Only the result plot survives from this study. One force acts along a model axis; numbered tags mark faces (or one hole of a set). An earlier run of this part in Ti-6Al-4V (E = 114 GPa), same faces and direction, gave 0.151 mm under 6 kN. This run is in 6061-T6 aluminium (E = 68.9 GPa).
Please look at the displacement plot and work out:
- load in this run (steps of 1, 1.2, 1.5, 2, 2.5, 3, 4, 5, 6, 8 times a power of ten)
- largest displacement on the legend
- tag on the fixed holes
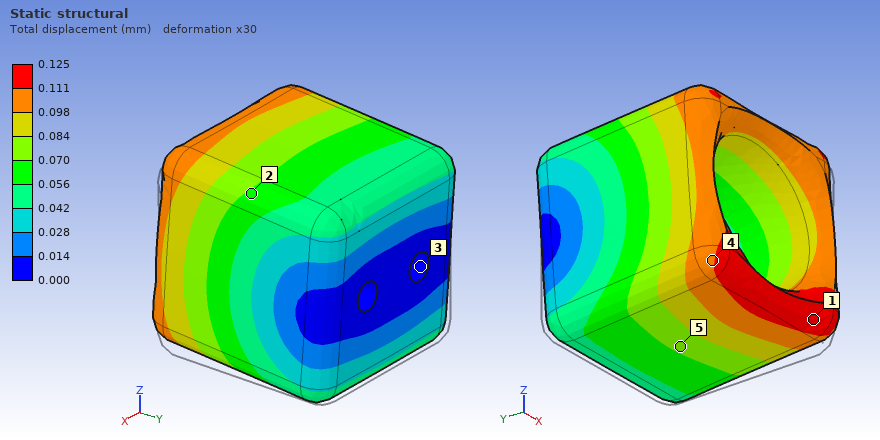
3 kN
0.125 mm
3
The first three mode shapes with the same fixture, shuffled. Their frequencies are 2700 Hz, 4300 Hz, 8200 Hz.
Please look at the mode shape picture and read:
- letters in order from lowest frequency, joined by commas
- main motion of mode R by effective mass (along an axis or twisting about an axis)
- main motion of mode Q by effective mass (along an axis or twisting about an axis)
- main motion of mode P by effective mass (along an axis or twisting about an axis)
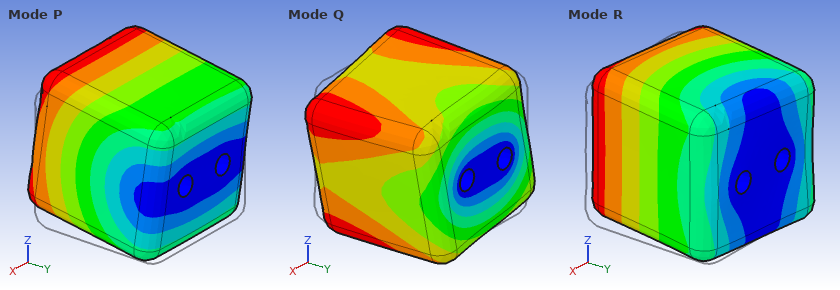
P, R, Q
along X
twisting about Y
along Z
